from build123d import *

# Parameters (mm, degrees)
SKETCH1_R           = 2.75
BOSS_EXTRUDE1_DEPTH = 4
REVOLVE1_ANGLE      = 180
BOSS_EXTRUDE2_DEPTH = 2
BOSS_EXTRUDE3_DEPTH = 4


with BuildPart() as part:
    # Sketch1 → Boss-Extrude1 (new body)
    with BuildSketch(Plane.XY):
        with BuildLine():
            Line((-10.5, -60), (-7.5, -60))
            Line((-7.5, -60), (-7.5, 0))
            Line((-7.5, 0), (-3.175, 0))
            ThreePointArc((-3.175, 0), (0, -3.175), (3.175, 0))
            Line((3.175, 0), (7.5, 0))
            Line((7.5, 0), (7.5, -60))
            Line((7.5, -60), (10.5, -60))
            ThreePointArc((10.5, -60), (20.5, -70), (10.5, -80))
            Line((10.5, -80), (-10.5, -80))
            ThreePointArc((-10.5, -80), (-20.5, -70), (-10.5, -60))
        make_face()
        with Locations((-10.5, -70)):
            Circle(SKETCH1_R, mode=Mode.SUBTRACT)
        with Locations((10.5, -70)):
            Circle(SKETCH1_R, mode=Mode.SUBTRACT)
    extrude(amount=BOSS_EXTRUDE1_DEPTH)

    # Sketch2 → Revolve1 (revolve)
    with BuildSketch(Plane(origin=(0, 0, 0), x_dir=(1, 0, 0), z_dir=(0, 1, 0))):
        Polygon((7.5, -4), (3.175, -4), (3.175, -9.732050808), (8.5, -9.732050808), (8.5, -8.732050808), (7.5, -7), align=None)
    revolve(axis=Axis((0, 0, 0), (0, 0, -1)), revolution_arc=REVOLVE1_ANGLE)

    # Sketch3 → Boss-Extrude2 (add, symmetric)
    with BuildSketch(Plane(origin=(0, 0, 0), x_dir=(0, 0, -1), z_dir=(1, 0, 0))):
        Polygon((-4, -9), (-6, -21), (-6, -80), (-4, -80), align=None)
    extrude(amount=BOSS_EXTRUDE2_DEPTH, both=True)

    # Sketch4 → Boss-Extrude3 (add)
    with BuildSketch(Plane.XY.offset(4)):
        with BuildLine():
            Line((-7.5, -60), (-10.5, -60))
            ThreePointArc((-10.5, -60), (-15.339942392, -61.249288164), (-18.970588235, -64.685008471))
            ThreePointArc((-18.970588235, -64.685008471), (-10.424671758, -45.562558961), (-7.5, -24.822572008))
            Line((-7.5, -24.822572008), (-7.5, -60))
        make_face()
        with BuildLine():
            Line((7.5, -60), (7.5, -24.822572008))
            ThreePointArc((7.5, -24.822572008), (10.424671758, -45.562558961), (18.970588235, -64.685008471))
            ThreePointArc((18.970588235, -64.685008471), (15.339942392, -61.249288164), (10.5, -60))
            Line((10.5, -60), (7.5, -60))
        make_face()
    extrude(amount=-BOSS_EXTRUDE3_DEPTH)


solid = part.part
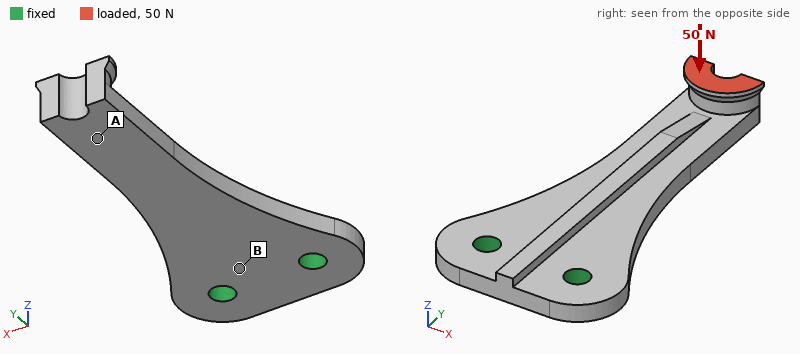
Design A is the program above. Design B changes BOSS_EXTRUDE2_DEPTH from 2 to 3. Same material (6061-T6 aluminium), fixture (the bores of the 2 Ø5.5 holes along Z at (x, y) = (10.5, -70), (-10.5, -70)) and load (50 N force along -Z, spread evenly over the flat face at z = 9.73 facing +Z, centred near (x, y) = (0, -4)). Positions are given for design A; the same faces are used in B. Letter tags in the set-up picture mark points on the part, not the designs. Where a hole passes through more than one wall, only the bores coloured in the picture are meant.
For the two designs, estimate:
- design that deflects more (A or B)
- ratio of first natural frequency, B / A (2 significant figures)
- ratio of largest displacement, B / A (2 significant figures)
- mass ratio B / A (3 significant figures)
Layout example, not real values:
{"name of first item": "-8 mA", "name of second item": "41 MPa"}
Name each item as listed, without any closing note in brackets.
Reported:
{"design that deflects more": "A", "ratio of first natural frequency, B / A": "1.1", "ratio of largest displacement, B / A": "0.88", "mass ratio B / A": "1.03"}
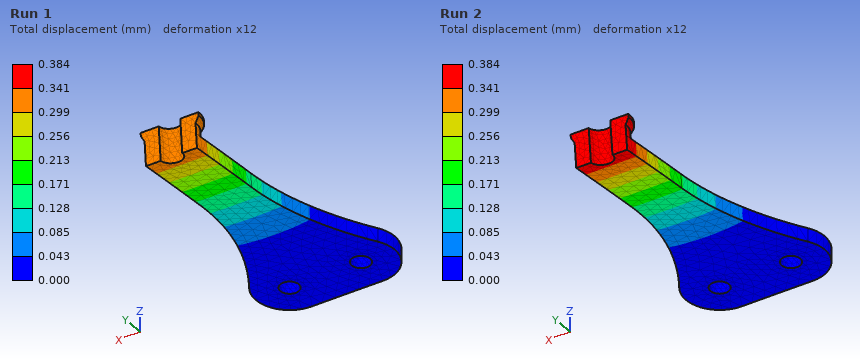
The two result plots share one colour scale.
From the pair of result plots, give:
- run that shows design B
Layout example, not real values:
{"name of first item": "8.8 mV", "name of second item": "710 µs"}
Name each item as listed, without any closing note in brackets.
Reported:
{"run that shows design B": "Run 1"}
